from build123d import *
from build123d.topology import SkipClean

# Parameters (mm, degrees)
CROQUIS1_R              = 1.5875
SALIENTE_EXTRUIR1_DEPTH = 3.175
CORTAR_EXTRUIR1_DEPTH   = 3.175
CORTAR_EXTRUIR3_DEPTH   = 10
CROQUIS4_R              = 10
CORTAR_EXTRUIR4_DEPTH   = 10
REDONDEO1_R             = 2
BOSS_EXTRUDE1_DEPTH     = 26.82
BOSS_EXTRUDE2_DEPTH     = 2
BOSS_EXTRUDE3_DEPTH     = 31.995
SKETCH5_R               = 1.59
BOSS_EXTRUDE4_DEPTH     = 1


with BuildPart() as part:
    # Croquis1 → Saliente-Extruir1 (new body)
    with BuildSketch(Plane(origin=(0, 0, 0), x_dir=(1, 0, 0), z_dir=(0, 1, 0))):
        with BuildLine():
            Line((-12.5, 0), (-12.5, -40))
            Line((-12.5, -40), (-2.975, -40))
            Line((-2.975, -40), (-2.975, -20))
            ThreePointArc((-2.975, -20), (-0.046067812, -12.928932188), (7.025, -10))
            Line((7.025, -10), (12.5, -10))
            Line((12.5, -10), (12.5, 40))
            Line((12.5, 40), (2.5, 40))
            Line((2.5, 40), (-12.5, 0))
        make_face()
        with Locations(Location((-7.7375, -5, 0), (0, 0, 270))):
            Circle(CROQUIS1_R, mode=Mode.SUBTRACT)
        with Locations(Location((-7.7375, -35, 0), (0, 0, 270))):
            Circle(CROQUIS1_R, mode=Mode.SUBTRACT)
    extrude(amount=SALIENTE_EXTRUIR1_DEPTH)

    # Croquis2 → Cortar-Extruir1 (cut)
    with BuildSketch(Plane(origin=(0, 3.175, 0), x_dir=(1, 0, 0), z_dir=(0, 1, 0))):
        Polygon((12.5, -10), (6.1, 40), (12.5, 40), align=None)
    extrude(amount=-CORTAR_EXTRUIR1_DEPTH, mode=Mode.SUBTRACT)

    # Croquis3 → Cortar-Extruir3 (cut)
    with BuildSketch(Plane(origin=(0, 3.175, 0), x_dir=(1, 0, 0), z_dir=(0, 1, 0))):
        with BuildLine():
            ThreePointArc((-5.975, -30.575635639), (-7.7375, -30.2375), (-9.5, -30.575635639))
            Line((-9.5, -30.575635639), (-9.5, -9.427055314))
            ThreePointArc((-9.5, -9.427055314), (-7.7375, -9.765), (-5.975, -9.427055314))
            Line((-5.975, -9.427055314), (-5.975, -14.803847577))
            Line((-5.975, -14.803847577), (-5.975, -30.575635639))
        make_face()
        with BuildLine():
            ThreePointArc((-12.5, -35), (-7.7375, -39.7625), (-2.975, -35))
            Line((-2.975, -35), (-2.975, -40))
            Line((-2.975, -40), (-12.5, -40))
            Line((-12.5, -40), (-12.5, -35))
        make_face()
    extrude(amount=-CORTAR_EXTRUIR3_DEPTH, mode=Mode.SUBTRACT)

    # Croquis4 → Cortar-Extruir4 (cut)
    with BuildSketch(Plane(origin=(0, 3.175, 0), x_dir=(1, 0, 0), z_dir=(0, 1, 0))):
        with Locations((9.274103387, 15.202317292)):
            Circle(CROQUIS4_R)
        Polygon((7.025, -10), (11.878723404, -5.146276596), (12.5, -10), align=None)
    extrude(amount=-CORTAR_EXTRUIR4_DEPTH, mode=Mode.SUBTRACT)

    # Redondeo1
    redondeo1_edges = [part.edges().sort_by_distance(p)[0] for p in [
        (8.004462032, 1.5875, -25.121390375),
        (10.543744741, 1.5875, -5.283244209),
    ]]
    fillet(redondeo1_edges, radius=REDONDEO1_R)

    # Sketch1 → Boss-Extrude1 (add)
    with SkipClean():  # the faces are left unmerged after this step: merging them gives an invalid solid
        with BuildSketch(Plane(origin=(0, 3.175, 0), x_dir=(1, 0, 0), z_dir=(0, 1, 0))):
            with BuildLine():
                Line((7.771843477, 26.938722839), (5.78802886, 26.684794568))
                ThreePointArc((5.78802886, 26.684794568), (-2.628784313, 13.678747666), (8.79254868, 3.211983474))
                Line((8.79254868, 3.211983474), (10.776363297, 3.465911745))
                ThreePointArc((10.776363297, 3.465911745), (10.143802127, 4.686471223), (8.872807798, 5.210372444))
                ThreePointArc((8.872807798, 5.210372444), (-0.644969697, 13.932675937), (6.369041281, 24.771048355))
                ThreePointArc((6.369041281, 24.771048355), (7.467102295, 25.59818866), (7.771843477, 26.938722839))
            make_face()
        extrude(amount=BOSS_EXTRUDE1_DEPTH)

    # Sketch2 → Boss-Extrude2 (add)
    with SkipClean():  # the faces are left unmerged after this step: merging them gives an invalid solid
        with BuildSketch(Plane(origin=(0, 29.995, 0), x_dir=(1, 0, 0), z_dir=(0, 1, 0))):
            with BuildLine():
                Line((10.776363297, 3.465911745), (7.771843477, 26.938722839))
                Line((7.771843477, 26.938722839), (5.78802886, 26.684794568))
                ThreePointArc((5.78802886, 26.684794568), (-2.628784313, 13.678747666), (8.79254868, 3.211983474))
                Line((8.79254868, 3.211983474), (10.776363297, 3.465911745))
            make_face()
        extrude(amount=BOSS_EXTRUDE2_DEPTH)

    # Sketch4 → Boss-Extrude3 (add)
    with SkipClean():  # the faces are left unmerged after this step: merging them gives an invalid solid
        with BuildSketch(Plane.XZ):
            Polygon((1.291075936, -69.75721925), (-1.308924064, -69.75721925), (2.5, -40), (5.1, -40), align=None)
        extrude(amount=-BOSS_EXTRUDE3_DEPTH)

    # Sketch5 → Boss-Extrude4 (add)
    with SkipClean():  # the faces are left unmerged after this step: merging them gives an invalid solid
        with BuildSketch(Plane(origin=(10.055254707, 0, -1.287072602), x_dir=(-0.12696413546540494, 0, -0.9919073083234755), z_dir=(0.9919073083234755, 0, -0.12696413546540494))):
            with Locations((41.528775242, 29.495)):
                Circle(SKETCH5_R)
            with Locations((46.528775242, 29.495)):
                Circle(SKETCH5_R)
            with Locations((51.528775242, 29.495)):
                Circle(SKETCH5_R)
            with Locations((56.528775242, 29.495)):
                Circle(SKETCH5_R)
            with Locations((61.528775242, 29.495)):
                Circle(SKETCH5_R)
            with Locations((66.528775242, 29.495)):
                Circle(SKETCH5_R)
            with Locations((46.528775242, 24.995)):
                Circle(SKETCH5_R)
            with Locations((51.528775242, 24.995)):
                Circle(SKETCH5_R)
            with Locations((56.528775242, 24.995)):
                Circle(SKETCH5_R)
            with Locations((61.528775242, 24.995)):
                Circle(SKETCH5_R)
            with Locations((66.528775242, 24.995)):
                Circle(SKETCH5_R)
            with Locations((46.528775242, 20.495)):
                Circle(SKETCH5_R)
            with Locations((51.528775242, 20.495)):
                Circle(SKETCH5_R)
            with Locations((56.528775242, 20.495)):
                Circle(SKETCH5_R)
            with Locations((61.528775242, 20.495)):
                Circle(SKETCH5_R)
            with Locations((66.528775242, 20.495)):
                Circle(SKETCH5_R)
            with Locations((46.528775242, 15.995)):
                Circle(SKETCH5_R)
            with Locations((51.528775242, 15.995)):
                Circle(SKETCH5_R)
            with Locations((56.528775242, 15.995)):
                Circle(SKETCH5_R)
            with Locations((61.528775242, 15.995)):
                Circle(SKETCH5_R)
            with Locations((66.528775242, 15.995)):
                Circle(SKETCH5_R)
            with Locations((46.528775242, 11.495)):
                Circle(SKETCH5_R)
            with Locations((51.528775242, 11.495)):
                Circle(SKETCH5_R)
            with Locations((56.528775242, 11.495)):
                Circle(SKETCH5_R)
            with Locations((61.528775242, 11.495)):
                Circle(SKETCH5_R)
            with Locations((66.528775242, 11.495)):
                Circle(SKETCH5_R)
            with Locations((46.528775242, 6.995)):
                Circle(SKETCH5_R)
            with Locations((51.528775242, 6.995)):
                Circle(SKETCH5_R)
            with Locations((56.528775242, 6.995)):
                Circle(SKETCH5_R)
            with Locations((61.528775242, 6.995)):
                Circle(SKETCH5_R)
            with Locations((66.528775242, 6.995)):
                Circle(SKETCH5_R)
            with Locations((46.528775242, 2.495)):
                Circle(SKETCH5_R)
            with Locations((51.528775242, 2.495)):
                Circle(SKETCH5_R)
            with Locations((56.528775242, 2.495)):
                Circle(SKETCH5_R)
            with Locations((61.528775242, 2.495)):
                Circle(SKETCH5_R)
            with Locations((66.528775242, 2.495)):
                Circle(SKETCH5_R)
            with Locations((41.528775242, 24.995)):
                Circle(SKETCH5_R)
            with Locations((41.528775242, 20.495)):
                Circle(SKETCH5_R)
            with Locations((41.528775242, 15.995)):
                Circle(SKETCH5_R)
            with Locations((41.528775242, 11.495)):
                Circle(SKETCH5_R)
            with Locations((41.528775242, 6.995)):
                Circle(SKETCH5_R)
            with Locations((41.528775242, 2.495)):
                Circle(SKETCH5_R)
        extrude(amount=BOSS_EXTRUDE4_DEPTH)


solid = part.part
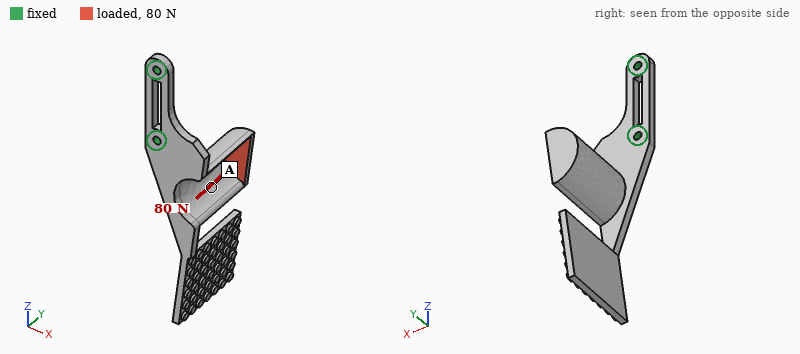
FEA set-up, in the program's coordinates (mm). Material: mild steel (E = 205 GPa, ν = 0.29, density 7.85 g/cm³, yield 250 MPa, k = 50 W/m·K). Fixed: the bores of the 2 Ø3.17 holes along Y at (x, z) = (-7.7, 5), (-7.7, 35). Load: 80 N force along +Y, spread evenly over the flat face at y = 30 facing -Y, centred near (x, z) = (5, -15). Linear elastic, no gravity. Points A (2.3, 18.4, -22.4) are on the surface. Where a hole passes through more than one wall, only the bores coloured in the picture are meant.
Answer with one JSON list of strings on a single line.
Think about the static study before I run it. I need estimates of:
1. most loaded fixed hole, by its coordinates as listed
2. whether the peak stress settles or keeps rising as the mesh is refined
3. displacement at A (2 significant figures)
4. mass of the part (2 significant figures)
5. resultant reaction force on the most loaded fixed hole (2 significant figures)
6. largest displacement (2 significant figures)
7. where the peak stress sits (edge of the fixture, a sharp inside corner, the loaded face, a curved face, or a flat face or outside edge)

["(-7.7, 5)", "keeps rising", "0.063 mm", "60 g", "91 N", "0.16 mm", "edge of the fixture"]
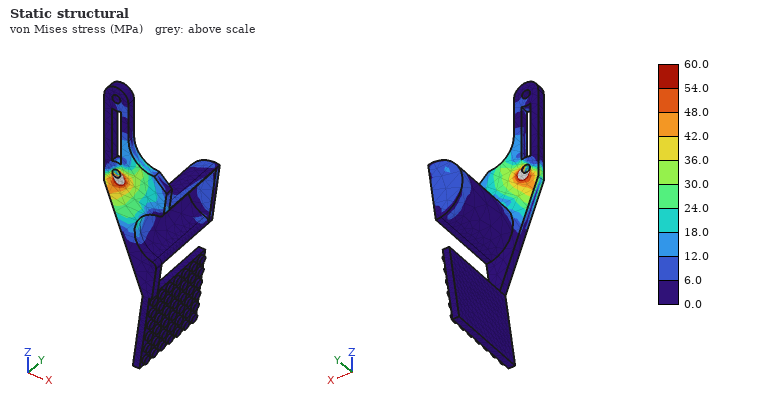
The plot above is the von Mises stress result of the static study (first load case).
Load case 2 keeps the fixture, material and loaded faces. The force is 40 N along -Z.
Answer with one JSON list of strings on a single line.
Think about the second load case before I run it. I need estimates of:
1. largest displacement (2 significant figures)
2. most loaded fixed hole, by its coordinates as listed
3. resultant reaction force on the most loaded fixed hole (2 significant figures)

["0.15 mm", "(-7.7, 5)", "30 N"]
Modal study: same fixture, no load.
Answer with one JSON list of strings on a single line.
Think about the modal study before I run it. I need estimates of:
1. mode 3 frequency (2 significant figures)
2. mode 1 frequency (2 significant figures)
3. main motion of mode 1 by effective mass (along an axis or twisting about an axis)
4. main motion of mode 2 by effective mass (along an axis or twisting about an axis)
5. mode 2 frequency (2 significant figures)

["1000 Hz", "310 Hz", "along Y", "along X", "440 Hz"]
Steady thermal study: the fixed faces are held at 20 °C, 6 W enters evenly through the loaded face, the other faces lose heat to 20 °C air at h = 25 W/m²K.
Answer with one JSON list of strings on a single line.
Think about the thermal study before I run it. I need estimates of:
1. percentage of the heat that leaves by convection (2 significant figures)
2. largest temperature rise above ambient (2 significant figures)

["54 %", "66 K"]
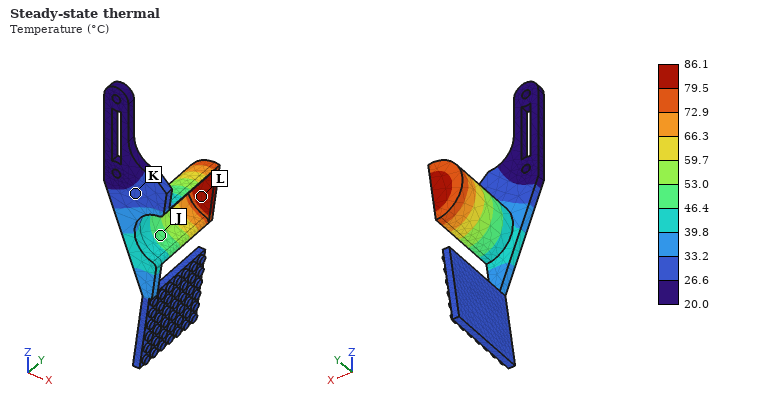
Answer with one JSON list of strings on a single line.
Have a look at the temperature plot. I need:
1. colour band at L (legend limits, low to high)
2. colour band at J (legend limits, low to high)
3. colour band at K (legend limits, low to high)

["79.5 to 86.1 °C", "46.4 to 53.0 °C", "26.6 to 33.2 °C"]
